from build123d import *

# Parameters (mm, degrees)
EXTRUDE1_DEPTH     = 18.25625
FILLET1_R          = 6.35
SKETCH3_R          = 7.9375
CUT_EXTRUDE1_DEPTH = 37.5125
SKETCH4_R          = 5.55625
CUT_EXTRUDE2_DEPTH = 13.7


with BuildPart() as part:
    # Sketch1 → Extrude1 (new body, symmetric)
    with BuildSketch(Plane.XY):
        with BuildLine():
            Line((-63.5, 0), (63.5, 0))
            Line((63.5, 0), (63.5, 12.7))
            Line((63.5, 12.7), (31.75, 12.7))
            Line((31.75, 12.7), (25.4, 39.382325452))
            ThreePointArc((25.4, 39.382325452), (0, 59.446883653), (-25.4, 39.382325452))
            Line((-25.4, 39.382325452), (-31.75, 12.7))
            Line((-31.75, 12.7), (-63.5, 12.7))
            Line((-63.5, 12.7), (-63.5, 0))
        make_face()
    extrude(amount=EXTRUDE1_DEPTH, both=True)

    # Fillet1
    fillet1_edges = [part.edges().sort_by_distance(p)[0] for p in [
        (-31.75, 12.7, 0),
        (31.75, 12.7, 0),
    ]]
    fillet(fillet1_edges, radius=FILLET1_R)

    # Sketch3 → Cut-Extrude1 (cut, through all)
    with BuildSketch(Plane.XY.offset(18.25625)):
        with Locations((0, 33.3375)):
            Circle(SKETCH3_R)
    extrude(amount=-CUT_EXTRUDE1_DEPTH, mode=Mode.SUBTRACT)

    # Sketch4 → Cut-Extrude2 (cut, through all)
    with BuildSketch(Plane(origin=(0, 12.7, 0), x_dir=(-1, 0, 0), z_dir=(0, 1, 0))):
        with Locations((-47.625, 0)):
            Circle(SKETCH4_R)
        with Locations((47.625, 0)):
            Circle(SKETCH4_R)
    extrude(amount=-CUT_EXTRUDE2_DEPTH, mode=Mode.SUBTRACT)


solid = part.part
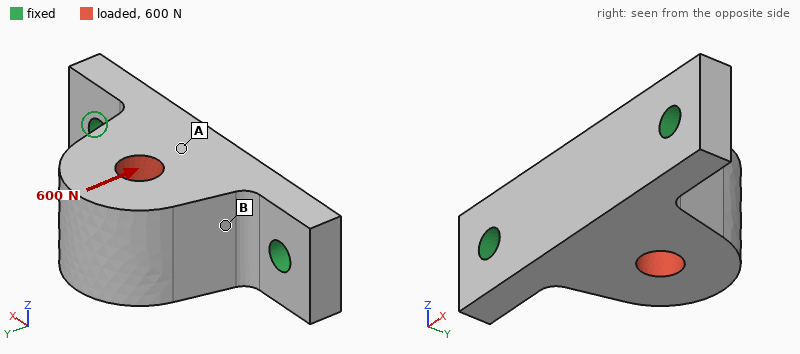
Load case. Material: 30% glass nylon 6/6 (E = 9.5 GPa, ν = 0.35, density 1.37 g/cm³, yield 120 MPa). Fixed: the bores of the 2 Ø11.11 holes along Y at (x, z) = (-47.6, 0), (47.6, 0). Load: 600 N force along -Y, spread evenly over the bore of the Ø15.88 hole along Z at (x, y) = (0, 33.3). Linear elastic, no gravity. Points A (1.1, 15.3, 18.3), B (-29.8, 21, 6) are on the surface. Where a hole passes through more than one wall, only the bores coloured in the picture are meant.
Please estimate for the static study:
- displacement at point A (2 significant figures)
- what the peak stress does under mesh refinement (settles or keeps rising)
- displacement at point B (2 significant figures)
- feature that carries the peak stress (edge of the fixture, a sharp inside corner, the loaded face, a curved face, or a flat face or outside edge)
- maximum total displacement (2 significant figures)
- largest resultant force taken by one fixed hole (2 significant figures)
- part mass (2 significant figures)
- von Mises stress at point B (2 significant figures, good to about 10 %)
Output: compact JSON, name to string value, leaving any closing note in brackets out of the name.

{"displacement at point A": "10 µm", "what the peak stress does under mesh refinement": "keeps rising", "displacement at point B": "7.5 µm", "feature that carries the peak stress": "edge of the fixture", "maximum total displacement": "10 µm", "largest resultant force taken by one fixed hole": "350 N", "part mass": "180 g", "von Mises stress at point B": "1.2 MPa"}
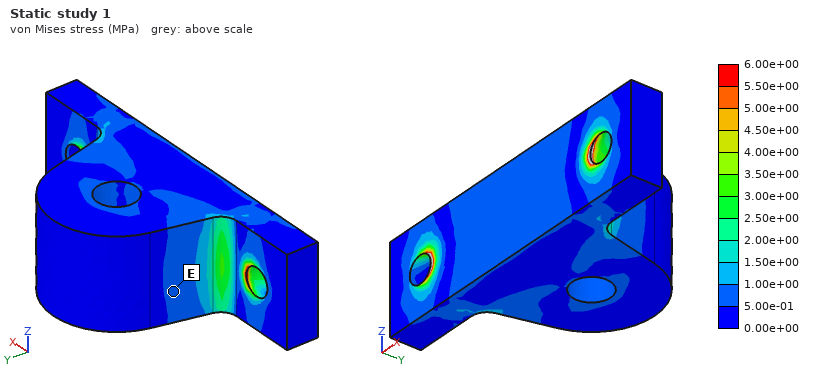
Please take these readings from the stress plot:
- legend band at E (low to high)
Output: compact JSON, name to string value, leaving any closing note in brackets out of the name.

{"legend band at E": "5.00e-01 to 1.00e+00 MPa"}
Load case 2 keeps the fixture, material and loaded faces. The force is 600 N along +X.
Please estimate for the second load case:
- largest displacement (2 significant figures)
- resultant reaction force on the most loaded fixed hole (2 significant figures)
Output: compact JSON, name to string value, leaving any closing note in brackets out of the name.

{"largest displacement": "9.9 µm", "resultant reaction force on the most loaded fixed hole": "360 N"}
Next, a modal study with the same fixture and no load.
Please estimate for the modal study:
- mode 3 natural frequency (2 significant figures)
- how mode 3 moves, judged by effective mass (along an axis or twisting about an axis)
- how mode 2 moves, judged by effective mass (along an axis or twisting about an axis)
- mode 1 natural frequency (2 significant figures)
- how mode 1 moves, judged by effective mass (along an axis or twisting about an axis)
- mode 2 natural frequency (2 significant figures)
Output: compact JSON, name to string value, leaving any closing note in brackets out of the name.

{"mode 3 natural frequency": "4200 Hz", "how mode 3 moves, judged by effective mass": "along X", "how mode 2 moves, judged by effective mass": "along Y", "mode 1 natural frequency": "1400 Hz", "how mode 1 moves, judged by effective mass": "along Z", "mode 2 natural frequency": "3400 Hz"}
